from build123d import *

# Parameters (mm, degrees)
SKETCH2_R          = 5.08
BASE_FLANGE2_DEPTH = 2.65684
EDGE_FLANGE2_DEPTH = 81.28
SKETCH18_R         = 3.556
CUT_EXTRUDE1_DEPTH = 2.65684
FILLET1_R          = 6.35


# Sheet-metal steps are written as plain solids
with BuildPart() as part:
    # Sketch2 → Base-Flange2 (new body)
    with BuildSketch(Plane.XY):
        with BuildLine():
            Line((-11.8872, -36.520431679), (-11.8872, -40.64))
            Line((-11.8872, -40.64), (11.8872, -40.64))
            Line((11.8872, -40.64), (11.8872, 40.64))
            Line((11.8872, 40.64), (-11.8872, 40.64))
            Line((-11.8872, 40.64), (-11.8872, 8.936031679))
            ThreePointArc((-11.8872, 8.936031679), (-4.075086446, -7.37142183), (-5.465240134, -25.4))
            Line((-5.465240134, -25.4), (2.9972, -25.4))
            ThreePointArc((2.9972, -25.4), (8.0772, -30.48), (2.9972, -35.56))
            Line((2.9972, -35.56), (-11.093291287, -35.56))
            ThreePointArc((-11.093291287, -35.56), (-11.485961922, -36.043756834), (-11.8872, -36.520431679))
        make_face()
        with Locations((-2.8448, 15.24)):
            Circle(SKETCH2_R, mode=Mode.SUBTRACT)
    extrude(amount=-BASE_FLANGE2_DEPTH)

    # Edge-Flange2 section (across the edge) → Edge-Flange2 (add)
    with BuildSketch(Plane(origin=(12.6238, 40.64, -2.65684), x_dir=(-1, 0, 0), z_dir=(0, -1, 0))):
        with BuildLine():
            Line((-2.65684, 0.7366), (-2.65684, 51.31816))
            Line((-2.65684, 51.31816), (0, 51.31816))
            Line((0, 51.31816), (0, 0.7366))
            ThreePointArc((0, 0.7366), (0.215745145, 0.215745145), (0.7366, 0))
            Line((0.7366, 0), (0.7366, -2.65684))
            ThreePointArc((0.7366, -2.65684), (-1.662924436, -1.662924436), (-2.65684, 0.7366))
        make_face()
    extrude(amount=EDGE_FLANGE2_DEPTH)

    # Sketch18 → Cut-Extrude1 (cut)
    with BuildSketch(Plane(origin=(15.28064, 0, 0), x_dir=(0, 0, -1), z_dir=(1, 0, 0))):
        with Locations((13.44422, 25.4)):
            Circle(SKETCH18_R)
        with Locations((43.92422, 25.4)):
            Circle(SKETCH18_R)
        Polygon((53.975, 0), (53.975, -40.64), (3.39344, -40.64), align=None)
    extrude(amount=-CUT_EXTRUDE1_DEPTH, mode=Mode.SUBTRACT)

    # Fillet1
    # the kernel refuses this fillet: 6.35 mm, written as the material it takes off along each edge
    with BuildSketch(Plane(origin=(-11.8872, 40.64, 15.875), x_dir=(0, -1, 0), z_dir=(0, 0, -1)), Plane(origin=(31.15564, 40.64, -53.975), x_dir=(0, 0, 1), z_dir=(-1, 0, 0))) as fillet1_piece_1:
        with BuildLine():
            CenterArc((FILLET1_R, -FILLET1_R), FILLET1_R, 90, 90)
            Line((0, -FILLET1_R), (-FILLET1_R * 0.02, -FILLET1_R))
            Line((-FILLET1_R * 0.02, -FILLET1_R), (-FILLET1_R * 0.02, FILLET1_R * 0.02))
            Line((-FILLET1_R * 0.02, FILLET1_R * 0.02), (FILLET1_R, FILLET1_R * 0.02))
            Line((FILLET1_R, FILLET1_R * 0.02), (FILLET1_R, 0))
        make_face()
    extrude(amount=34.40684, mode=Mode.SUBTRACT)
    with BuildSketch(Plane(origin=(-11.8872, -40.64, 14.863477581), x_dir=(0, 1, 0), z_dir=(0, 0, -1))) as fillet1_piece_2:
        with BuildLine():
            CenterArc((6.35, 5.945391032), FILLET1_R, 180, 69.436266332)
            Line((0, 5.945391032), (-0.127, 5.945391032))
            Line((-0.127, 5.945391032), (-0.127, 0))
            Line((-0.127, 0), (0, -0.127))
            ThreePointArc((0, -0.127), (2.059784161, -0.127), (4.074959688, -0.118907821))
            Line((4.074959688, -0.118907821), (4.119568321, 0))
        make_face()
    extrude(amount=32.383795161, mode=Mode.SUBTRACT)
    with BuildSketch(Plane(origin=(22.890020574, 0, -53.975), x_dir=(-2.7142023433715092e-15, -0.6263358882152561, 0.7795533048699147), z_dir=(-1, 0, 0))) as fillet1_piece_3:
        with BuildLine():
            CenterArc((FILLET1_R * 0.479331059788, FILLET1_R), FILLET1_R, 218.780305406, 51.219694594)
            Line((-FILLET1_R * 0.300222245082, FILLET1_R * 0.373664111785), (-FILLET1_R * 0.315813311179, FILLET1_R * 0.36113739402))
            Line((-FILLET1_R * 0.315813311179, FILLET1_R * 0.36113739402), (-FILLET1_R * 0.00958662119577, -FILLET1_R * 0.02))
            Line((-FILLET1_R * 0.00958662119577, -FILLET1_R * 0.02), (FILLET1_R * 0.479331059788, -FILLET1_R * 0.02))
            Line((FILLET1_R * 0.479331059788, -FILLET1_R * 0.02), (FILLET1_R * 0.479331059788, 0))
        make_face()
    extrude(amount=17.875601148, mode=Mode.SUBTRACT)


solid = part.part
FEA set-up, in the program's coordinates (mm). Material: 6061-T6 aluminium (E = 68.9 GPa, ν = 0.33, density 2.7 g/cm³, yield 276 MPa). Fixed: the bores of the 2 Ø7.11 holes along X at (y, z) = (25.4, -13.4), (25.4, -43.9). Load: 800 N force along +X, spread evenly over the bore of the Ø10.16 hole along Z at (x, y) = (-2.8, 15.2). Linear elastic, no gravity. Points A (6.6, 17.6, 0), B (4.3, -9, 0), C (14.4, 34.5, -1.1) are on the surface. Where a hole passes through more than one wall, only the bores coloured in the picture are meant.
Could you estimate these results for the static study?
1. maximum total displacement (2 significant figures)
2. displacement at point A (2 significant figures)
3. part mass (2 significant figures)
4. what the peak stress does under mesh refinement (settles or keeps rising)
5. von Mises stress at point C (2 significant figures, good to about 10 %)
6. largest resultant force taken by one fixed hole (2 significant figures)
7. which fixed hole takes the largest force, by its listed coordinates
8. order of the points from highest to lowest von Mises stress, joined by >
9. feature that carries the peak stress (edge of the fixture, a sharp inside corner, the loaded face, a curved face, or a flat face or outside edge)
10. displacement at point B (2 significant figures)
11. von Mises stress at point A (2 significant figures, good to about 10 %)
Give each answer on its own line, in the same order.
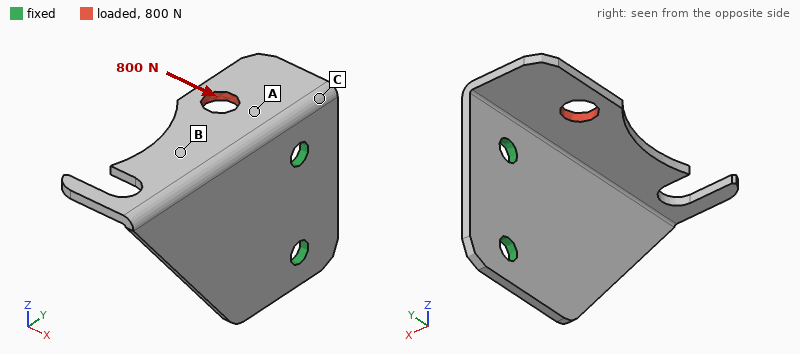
0.77 mm
0.21 mm
34 g
keeps rising
63 MPa
860 N
(25.4, -13.4)
C > A > B
edge of the fixture
0.44 mm
34 MPa
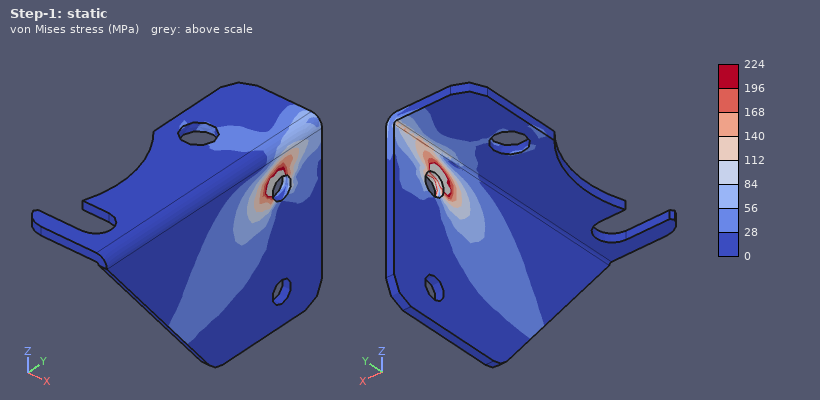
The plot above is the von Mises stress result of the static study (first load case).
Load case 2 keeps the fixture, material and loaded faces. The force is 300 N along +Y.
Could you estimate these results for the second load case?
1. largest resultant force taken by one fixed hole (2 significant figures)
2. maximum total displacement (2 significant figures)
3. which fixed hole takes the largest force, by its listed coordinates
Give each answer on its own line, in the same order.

380 N
0.42 mm
(25.4, -13.4)
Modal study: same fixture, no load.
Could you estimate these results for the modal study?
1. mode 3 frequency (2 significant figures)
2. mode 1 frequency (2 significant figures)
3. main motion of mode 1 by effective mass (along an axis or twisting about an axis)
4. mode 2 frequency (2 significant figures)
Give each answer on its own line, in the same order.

2700 Hz
980 Hz
along X
1900 Hz
